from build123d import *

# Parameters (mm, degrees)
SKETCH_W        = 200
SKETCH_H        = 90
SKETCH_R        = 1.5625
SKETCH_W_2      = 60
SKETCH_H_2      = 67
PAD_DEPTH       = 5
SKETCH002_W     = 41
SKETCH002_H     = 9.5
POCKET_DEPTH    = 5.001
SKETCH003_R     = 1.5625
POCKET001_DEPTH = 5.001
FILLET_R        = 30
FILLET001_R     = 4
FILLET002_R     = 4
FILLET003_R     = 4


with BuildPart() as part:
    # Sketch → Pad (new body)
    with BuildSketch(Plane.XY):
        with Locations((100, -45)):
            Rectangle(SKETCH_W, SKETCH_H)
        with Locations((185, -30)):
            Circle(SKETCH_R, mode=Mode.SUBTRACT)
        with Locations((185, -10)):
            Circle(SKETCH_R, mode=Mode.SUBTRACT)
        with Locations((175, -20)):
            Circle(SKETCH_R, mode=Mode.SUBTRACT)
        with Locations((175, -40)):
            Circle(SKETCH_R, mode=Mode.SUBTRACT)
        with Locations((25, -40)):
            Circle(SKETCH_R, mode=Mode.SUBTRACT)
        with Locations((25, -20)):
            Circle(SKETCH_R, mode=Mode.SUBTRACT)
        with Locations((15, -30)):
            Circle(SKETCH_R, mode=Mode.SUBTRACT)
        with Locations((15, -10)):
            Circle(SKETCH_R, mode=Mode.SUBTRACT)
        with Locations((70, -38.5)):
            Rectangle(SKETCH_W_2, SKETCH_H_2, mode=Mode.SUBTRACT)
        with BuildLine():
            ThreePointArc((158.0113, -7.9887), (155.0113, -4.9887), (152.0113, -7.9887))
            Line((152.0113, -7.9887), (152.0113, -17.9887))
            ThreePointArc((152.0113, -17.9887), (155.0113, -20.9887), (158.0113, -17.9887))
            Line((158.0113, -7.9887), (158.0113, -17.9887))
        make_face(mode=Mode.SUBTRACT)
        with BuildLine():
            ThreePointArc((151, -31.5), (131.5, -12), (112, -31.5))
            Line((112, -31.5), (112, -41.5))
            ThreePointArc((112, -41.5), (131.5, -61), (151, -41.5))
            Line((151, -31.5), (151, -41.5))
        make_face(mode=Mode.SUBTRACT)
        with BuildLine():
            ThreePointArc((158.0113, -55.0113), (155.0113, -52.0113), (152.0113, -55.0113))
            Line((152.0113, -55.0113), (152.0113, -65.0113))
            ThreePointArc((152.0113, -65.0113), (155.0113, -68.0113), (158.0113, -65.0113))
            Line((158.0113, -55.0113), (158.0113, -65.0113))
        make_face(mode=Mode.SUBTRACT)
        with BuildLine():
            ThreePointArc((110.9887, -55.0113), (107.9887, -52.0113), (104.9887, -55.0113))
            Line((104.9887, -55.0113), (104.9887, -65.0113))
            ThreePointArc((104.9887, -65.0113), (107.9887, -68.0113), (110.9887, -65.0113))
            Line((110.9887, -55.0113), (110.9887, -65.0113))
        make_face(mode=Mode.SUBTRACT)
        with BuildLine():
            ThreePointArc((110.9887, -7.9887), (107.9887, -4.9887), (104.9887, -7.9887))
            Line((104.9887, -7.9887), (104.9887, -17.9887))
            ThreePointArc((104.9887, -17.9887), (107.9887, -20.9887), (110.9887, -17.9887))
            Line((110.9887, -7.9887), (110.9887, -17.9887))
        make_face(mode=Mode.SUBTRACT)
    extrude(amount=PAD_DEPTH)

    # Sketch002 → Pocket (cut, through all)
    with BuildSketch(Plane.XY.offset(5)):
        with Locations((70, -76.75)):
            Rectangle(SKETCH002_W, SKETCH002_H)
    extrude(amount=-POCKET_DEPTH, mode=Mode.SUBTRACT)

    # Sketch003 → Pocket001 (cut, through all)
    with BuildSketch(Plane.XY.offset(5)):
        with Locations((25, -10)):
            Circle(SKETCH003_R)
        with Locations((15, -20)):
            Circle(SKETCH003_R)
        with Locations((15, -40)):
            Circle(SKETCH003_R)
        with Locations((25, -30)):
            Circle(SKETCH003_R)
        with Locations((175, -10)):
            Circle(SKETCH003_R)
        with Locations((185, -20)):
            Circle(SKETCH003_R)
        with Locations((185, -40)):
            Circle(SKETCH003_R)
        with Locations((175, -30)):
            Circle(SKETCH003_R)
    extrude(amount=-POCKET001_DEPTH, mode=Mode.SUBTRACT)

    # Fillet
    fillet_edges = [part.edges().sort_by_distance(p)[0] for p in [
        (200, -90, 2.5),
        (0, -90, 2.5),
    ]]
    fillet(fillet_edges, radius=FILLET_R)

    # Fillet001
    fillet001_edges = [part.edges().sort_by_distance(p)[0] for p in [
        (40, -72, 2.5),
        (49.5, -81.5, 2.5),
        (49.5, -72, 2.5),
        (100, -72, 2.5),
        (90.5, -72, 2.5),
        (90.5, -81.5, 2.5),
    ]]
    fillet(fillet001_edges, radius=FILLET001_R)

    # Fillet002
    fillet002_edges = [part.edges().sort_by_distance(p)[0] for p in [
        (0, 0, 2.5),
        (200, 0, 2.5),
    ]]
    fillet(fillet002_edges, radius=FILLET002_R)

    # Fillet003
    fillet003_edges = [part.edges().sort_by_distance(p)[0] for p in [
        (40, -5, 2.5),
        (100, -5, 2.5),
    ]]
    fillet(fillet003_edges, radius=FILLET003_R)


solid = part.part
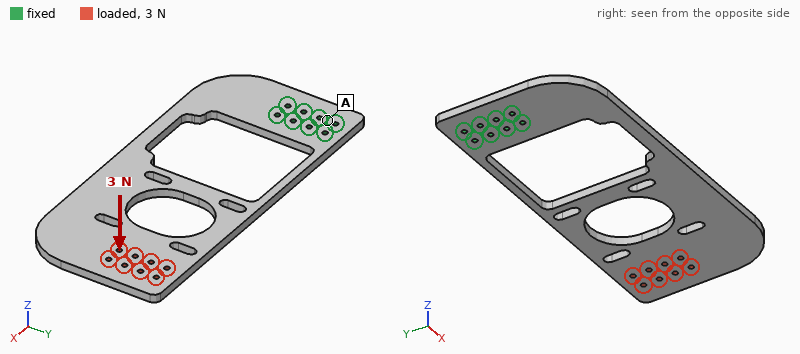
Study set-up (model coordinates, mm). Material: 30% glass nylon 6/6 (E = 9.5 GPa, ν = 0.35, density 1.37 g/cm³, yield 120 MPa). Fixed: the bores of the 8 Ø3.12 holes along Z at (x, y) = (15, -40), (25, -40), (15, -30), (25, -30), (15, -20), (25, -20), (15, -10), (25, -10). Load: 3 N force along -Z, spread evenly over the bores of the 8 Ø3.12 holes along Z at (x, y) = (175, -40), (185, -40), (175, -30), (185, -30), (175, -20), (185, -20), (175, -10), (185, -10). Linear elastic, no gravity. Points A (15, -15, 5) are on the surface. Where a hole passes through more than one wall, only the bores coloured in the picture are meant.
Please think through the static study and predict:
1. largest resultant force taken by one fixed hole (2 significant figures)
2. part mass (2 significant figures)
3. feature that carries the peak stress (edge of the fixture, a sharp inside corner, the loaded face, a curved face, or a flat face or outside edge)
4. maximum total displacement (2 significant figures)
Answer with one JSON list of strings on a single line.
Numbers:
["15 N", "76 g", "a curved face", "2.6 mm"]
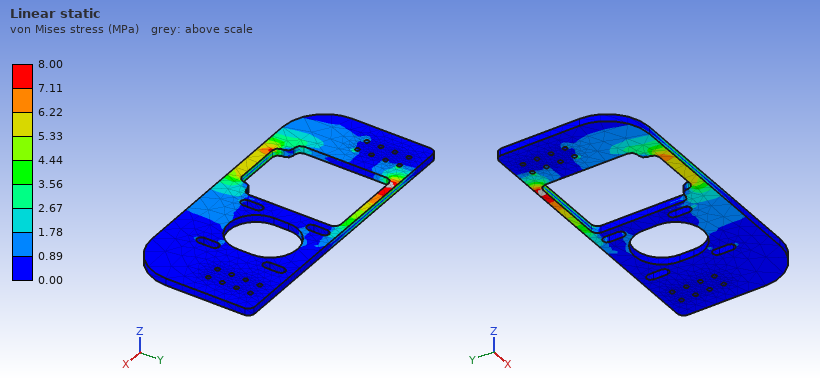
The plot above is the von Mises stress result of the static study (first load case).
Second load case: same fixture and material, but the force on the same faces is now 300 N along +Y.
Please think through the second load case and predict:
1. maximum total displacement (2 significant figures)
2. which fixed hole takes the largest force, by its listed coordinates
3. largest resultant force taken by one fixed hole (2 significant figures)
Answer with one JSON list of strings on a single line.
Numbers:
["2.4 mm", "(25, -40)", "1.1 kN"]
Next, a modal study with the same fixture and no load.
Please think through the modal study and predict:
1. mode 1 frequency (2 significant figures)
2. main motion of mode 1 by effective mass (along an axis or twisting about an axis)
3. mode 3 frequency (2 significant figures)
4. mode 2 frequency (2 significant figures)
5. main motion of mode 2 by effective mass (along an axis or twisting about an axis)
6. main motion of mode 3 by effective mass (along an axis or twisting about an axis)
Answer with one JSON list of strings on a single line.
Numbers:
["34 Hz", "along Z", "280 Hz", "170 Hz", "twisting about X", "along Y"]
